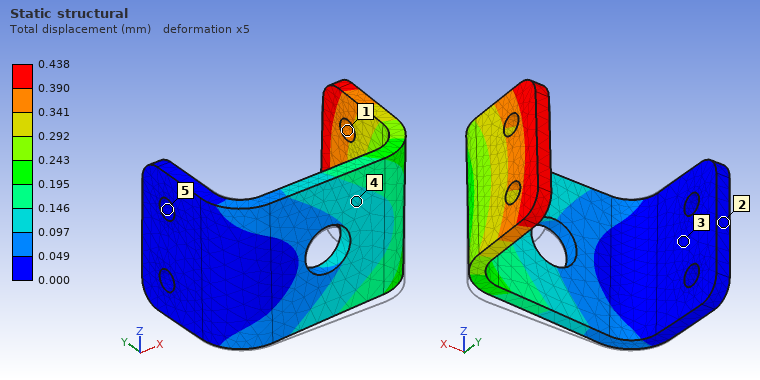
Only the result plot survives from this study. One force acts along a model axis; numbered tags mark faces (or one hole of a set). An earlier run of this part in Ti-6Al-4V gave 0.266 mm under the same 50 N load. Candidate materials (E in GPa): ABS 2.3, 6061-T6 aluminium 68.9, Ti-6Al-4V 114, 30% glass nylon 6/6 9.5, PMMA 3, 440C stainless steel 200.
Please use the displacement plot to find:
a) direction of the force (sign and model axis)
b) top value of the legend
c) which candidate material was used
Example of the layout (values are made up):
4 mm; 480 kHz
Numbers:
+Z; 0.438 mm; 6061-T6 aluminium
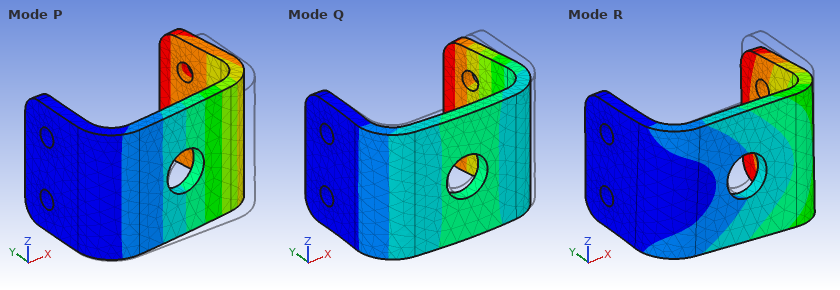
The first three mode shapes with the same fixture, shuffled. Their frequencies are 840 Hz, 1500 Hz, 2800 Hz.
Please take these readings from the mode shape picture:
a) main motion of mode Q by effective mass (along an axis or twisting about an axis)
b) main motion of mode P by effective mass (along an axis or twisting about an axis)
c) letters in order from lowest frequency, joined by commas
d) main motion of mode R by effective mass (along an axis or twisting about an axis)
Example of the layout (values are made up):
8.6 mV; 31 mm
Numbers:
along X; along Y; P, R, Q; along Z
